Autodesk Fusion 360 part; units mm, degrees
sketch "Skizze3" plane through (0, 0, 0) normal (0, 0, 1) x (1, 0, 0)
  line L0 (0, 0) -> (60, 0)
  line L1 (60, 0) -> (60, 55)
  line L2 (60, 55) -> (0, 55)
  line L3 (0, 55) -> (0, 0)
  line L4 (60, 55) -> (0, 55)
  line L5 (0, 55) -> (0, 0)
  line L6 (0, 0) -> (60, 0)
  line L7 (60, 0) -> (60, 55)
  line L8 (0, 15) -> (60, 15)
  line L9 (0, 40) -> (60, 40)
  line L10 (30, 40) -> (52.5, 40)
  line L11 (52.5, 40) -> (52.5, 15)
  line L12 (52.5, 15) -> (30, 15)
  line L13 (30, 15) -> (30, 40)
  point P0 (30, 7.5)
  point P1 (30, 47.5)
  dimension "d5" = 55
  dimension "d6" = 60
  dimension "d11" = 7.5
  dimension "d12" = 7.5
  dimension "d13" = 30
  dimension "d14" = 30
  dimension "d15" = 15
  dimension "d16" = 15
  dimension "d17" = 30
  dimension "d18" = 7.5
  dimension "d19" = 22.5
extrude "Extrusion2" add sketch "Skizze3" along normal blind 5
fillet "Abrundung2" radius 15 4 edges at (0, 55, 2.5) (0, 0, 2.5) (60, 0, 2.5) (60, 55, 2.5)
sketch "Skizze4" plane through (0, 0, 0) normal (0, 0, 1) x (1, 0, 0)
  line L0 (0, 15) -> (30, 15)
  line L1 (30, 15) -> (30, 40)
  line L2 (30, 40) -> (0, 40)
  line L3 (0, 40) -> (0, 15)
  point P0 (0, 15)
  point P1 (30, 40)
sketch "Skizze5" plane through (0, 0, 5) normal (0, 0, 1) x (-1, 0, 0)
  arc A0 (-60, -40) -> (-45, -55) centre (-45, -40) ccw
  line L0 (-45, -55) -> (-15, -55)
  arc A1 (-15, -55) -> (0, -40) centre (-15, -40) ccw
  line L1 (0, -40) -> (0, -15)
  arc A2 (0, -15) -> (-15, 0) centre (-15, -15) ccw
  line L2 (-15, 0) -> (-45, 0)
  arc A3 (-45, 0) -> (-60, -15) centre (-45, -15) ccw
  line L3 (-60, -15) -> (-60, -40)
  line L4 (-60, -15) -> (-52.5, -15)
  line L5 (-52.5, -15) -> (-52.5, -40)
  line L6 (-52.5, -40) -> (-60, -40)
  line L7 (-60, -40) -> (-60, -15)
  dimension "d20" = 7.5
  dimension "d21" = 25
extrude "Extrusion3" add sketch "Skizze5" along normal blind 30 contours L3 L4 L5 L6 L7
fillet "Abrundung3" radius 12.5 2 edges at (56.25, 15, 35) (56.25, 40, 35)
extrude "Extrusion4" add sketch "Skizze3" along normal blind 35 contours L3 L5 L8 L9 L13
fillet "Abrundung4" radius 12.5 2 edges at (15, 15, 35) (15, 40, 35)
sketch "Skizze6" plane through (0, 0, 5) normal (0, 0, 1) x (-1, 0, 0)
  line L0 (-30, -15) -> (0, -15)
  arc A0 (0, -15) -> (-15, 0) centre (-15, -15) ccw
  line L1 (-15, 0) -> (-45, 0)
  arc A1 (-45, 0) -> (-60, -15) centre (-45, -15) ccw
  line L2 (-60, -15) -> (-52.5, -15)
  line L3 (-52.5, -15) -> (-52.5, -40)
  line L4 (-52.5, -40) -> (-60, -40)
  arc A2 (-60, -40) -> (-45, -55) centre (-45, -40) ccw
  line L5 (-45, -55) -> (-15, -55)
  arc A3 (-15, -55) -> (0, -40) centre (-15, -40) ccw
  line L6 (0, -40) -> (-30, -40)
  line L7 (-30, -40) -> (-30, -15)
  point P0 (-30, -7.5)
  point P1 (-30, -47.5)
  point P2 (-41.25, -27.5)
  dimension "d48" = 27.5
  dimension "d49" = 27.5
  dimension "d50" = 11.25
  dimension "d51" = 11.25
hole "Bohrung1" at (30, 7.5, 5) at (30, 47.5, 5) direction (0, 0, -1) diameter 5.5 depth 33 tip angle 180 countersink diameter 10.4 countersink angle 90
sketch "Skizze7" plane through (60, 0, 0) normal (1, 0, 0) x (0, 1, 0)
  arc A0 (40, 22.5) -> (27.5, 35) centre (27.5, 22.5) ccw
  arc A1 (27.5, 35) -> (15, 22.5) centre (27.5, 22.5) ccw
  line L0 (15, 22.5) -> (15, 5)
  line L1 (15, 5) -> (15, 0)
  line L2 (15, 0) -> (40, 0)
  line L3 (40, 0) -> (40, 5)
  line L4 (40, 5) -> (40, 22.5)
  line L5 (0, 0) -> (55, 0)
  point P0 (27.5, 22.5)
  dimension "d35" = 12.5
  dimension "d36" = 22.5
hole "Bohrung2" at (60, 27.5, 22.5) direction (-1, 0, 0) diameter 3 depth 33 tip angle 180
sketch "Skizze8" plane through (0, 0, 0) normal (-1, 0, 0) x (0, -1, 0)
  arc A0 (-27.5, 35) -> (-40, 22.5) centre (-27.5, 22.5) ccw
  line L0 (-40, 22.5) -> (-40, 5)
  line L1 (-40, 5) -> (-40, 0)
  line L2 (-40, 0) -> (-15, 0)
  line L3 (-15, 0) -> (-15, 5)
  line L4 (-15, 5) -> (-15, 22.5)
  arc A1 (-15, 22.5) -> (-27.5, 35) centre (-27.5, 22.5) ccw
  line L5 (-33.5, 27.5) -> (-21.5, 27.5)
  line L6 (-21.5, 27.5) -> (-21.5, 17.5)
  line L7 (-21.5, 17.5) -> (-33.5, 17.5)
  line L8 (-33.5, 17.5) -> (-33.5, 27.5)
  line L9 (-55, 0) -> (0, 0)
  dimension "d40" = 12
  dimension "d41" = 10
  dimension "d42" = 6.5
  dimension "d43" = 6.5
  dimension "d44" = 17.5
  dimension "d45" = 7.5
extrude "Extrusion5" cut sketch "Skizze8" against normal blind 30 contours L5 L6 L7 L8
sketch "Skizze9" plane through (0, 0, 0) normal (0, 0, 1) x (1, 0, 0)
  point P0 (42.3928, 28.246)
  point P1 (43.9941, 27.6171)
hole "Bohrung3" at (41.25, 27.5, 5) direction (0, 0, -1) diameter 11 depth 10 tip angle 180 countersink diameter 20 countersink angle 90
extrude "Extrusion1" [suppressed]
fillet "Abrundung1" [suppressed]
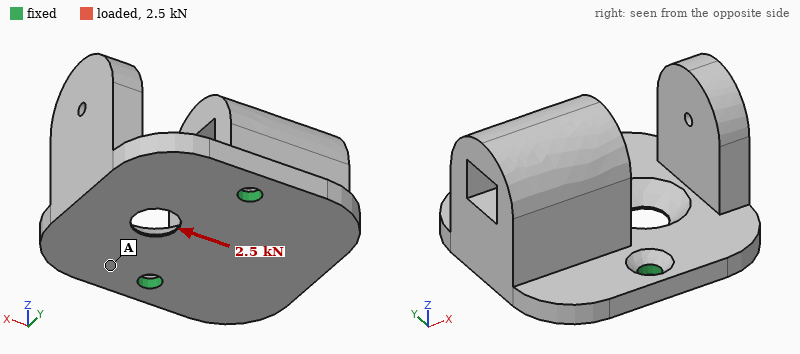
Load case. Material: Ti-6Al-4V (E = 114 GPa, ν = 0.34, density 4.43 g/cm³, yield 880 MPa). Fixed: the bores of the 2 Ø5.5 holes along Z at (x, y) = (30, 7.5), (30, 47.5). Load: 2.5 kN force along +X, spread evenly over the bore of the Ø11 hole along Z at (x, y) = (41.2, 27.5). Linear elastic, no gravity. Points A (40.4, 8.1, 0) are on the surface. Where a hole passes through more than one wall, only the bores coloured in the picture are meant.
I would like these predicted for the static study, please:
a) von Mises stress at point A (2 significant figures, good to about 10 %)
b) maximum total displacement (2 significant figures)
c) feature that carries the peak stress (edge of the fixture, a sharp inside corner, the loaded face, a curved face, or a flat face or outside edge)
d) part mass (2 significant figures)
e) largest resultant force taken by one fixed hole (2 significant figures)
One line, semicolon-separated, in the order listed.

24 MPa; 50 µm; the loaded face; 160 g; 1.3 kN
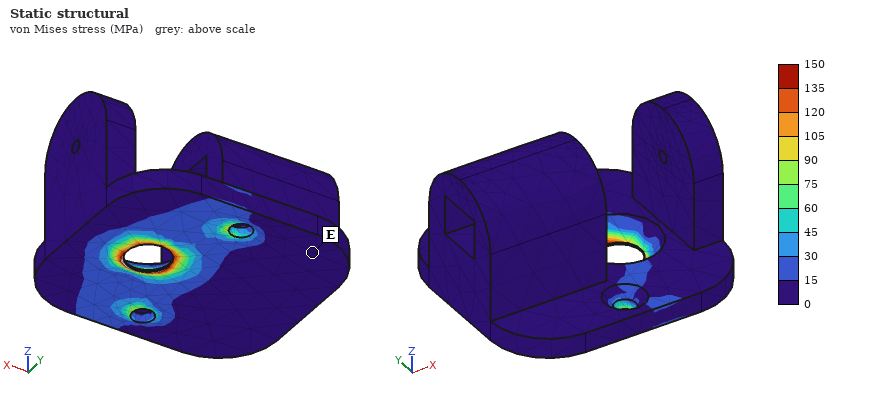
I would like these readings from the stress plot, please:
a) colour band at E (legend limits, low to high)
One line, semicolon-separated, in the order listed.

0 to 15 MPa
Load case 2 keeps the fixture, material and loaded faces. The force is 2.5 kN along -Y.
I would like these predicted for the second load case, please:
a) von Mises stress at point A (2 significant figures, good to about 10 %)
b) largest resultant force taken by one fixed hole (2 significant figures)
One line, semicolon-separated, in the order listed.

19 MPa; 1.4 kN
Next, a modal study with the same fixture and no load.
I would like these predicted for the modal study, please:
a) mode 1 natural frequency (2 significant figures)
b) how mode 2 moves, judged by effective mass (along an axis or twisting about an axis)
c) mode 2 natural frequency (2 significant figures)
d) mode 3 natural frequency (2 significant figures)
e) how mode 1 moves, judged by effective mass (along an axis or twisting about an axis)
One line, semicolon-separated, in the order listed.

1400 Hz; along Z; 2000 Hz; 3700 Hz; along X
